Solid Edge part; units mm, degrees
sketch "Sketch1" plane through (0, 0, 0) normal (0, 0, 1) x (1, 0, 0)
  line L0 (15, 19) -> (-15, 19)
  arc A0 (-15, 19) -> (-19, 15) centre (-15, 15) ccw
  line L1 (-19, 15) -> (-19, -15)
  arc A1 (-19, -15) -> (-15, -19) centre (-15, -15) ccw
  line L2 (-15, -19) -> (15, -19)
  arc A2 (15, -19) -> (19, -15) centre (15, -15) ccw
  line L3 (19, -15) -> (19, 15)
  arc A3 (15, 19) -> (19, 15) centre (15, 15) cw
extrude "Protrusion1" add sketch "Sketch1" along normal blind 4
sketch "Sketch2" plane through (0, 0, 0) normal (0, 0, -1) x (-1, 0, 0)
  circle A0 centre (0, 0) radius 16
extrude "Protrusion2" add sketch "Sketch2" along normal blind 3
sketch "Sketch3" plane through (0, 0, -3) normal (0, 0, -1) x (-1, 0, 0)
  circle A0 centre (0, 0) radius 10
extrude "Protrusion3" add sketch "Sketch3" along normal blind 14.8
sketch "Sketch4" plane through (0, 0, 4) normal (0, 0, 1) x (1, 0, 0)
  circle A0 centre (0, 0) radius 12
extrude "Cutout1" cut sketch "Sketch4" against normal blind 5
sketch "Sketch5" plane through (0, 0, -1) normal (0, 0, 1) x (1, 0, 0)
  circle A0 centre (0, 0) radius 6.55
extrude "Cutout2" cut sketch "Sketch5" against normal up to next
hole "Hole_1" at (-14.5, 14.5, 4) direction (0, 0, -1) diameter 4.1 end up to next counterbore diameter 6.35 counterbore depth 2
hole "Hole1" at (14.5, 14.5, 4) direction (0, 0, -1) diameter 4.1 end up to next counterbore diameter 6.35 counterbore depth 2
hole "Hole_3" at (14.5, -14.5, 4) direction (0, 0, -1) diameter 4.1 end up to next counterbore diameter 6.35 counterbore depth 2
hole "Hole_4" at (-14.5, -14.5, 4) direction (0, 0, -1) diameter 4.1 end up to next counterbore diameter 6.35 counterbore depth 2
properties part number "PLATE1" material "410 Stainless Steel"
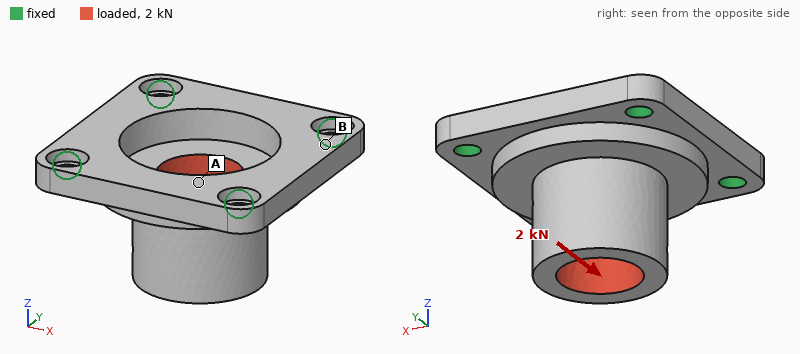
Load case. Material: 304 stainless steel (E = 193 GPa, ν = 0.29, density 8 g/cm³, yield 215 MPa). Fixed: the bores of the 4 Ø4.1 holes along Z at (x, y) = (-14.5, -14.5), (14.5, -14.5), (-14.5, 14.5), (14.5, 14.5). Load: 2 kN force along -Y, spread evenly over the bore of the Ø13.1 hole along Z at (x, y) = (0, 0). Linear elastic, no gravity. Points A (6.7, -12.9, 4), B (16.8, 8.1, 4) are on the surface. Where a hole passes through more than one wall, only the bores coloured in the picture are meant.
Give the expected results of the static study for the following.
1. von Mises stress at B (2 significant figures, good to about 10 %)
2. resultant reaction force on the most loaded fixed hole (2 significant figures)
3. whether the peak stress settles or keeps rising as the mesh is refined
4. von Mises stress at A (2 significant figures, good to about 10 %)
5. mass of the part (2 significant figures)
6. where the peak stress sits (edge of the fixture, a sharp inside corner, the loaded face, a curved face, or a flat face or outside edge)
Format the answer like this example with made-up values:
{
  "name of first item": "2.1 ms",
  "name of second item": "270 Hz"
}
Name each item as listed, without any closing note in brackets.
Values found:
{
  "von Mises stress at B": "9.5 MPa",
  "resultant reaction force on the most loaded fixed hole": "660 N",
  "whether the peak stress settles or keeps rising as the mesh is refined": "keeps rising",
  "von Mises stress at A": "16 MPa",
  "mass of the part": "63 g",
  "where the peak stress sits": "edge of the fixture"
}
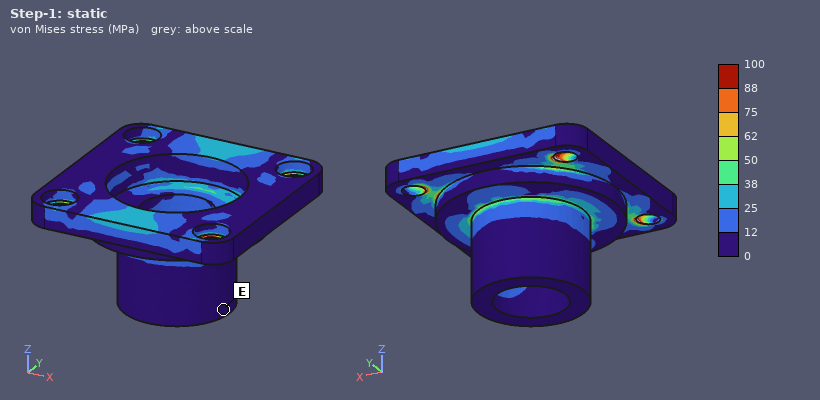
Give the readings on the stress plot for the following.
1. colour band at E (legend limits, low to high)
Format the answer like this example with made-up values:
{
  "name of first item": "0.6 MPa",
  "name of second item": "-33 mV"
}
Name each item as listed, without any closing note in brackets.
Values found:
{
  "colour band at E": "0 to 12 MPa"
}
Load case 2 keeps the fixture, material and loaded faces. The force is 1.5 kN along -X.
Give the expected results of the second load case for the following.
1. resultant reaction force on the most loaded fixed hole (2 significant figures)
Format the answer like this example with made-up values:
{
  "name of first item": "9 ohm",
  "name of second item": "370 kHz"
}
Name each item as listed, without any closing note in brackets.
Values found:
{
  "resultant reaction force on the most loaded fixed hole": "490 N"
}
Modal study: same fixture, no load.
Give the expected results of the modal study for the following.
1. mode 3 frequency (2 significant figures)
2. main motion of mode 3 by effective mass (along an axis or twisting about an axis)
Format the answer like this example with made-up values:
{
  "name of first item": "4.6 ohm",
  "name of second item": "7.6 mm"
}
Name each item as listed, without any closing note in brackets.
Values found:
{
  "mode 3 frequency": "14 kHz",
  "main motion of mode 3 by effective mass": "along Z"
}
